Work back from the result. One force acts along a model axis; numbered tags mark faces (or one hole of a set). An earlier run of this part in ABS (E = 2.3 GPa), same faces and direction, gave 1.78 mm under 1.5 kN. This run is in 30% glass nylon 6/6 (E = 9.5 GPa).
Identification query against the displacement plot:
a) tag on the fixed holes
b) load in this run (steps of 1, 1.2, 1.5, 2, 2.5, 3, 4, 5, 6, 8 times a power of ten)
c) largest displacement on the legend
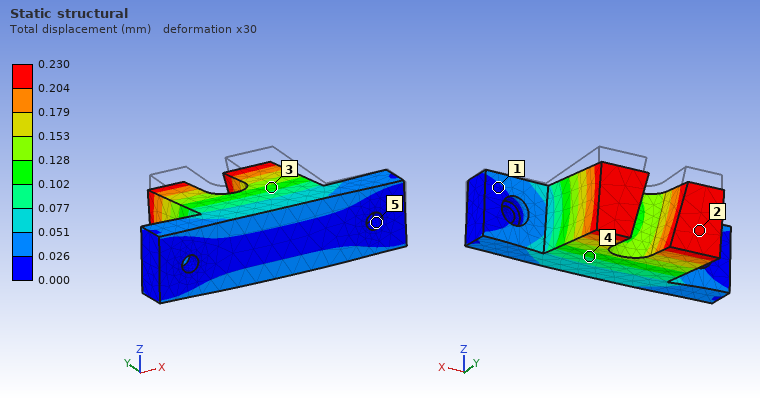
5
800 N
0.230 mm
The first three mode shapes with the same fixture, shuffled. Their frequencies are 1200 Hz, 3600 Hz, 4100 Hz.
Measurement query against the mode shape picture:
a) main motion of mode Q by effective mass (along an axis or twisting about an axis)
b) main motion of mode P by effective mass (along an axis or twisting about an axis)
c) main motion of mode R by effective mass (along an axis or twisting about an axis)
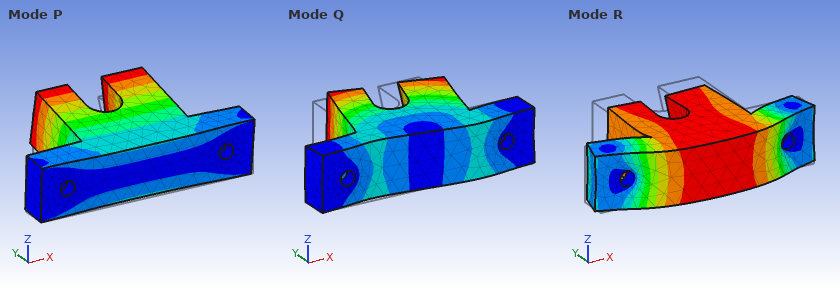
along X
along Z
along Y
